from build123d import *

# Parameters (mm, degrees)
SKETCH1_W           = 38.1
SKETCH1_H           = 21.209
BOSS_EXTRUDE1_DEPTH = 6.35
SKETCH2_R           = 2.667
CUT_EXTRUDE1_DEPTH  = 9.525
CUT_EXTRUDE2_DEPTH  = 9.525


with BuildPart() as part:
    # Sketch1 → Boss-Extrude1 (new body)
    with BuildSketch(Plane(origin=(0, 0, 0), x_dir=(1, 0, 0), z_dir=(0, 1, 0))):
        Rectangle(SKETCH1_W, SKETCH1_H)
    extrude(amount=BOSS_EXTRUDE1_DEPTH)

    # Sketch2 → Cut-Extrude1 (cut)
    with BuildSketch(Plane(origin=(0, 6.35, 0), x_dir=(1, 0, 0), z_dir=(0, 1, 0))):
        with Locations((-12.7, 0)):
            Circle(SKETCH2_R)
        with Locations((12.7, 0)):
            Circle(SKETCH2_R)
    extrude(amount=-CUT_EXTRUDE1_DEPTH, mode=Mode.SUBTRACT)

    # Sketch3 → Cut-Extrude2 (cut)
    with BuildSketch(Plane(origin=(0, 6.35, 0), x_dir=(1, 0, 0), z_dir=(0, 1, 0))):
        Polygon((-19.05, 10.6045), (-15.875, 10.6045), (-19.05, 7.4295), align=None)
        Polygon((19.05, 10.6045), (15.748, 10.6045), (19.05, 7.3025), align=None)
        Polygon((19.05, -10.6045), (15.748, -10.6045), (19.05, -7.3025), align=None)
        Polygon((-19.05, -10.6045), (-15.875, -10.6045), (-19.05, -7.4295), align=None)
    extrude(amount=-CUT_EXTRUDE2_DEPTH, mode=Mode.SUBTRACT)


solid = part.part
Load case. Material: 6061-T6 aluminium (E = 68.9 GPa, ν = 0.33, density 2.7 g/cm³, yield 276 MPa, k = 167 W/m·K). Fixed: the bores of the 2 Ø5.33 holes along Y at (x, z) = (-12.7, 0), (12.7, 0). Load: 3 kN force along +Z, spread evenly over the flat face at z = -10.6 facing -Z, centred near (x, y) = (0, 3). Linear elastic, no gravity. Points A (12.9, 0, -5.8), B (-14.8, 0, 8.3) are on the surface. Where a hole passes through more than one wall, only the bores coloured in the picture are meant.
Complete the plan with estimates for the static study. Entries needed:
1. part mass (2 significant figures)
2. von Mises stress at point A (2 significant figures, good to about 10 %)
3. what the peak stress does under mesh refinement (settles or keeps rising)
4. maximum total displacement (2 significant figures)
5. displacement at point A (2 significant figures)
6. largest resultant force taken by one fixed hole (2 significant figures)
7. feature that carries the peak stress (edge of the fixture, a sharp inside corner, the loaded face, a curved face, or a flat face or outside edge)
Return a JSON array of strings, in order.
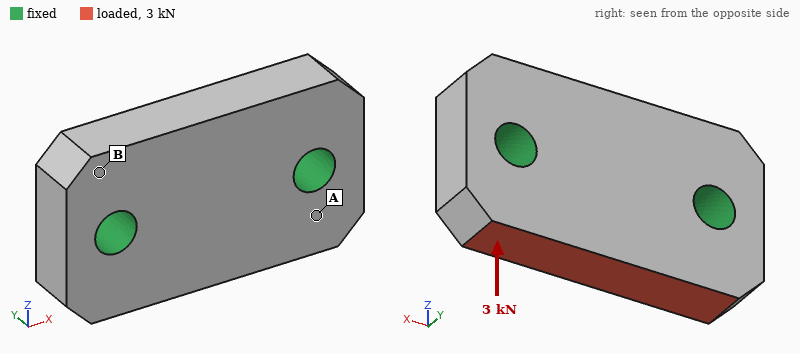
["13 g", "17 MPa", "keeps rising", "4.2 µm", "0.90 µm", "1.5 kN", "edge of the fixture"]
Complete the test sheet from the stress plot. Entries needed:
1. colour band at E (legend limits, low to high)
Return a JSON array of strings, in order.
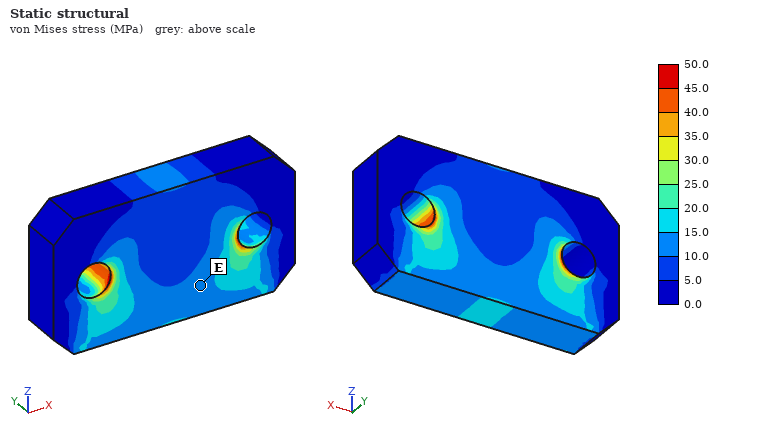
["10.0 to 15.0 MPa"]
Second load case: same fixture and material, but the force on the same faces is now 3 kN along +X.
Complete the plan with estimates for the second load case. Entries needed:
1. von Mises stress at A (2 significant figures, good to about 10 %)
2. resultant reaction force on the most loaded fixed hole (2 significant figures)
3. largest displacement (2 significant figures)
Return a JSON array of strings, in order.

["20 MPa", "1.8 kN", "7.1 µm"]
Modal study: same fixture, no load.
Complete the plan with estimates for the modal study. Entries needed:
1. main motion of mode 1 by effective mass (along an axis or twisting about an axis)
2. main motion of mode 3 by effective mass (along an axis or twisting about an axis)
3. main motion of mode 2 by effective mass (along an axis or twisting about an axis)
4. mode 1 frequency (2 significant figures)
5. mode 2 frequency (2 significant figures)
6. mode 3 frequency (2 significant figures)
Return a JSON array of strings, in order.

["twisting about X", "along Z", "along Y", "32 kHz", "35 kHz", "51 kHz"]
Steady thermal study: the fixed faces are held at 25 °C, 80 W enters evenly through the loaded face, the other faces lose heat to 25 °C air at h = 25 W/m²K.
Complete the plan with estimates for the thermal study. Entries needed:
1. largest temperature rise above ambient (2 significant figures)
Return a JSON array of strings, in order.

["28 K"]
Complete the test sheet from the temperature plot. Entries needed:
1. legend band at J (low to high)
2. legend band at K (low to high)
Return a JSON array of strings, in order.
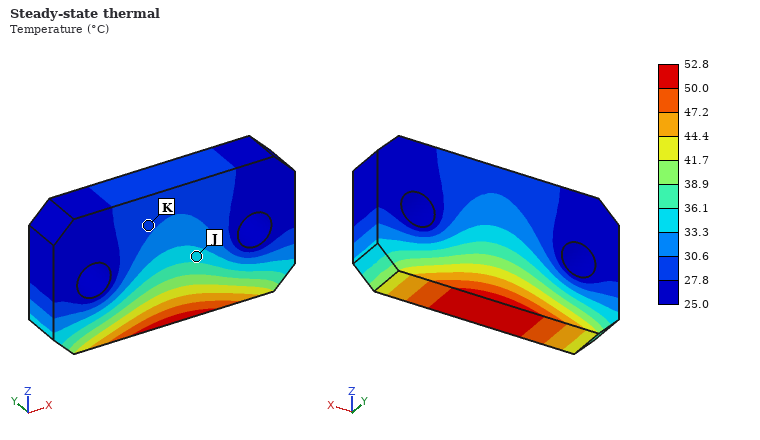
["33.3 to 36.1 °C", "27.8 to 30.6 °C"]
